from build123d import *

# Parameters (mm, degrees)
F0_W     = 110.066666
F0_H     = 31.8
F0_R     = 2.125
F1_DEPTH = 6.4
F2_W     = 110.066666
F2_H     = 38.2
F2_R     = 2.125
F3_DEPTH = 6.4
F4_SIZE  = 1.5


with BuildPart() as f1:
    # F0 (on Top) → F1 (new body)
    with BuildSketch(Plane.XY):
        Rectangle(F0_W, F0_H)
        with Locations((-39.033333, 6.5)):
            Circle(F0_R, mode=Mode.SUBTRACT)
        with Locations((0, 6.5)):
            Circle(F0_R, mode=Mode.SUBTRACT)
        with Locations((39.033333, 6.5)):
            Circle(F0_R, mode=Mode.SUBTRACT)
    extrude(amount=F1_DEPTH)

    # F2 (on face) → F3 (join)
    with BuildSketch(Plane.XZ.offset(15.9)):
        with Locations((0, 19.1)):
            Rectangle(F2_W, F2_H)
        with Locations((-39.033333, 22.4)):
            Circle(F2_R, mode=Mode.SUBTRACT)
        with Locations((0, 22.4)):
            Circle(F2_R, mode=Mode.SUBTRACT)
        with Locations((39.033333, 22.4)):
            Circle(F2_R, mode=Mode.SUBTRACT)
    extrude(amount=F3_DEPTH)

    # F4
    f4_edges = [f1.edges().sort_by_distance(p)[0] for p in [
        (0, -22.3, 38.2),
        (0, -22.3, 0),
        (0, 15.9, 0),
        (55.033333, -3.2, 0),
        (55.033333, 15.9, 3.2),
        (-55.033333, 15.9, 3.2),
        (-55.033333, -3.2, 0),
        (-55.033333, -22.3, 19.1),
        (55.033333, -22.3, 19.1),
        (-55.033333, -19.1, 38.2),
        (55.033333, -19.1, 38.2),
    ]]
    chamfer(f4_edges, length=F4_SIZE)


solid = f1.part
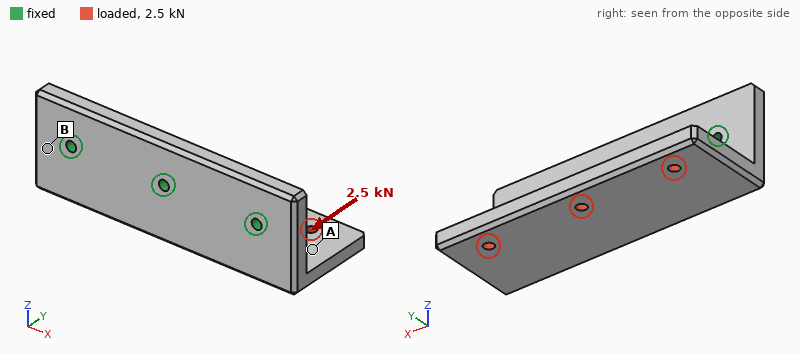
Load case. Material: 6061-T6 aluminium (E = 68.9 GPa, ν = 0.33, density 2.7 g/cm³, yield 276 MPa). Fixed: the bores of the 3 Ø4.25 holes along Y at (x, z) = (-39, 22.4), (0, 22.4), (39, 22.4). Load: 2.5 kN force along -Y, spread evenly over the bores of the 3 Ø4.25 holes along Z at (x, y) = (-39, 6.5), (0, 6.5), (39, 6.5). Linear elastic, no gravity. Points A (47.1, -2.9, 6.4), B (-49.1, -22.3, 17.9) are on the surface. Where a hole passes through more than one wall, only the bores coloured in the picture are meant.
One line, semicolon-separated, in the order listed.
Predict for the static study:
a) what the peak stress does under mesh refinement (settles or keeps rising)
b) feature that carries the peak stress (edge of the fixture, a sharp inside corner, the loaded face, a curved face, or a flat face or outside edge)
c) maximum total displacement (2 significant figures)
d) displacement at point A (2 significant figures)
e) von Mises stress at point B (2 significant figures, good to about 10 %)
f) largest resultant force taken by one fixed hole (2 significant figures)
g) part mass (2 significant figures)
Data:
keeps rising; edge of the fixture; 0.14 mm; 0.075 mm; 35 MPa; 850 N; 130 g
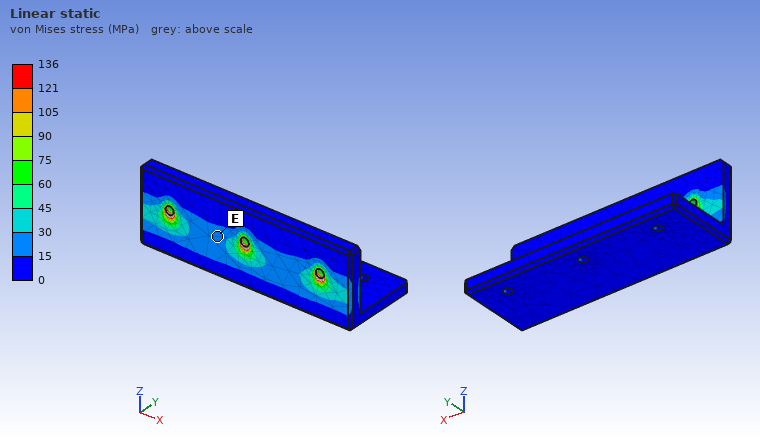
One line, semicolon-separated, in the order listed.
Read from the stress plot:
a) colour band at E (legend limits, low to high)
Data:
15 to 30 MPa
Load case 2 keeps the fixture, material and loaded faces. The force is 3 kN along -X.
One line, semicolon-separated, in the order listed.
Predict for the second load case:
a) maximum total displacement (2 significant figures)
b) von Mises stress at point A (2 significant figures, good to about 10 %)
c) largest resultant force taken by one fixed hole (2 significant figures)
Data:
96 µm; 15 MPa; 1.5 kN
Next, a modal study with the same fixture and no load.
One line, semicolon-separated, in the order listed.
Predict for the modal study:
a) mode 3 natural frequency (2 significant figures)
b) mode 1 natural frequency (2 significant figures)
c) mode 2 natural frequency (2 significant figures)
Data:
6000 Hz; 2200 Hz; 3200 Hz
